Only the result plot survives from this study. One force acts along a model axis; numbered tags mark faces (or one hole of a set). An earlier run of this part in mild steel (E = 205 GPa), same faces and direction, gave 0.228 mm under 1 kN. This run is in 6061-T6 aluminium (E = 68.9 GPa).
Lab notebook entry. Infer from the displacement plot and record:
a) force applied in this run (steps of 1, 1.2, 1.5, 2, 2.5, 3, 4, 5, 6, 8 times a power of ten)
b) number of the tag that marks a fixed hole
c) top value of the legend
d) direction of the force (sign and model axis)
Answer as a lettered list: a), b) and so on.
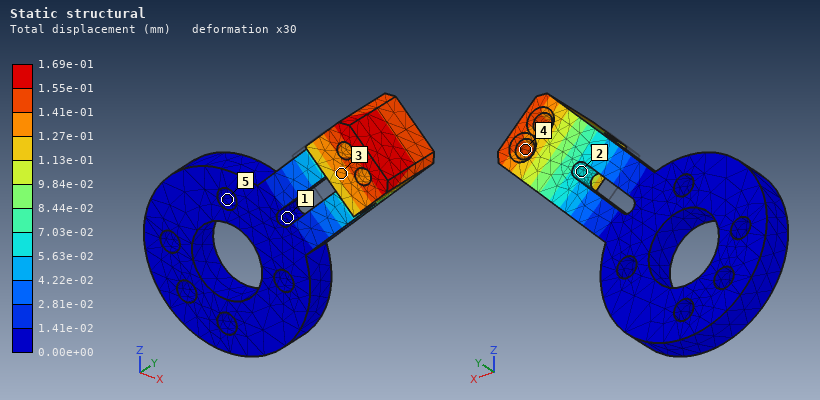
a) 250 N
b) 5
c) 1.69e-01 mm
d) +Y
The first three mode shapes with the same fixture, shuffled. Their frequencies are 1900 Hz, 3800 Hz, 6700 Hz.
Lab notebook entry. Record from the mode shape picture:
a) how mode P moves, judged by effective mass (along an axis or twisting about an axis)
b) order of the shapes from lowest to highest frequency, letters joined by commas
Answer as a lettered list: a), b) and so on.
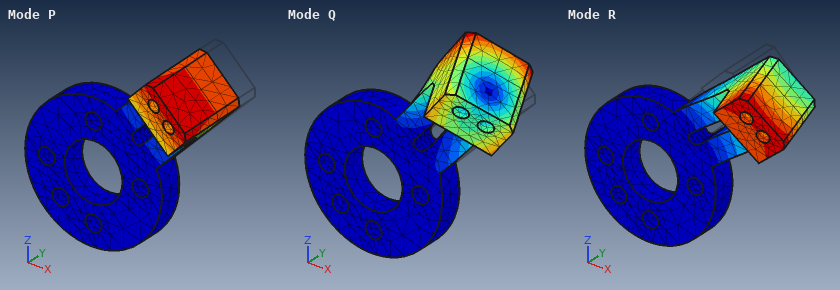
a) along Y
b) P, R, Q
